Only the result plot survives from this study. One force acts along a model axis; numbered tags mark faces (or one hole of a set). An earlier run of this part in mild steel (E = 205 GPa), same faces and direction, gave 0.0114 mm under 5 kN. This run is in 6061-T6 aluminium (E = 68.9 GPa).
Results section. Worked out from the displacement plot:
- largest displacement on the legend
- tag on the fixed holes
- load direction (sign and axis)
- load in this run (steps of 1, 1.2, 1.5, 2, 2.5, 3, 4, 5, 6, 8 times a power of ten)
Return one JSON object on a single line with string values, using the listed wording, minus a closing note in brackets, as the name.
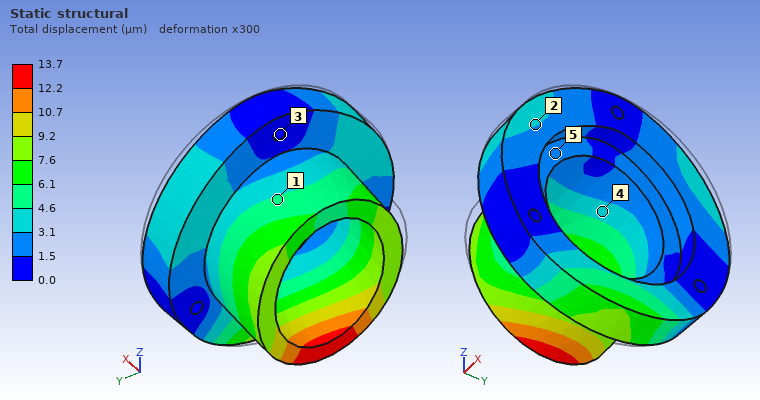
{"largest displacement on the legend": "13.7 µm", "tag on the fixed holes": "3", "load direction": "-Z", "load in this run": "2 kN"}
